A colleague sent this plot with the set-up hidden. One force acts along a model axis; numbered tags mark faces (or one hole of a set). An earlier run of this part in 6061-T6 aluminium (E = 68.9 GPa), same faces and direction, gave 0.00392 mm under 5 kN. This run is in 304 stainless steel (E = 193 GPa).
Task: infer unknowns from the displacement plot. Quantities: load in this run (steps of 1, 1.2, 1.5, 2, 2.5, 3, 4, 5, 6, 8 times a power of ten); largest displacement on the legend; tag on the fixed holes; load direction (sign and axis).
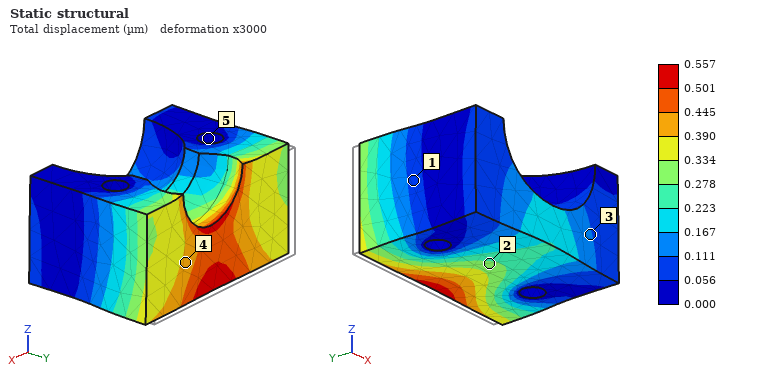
2 kN
0.557 µm
5
-Y
